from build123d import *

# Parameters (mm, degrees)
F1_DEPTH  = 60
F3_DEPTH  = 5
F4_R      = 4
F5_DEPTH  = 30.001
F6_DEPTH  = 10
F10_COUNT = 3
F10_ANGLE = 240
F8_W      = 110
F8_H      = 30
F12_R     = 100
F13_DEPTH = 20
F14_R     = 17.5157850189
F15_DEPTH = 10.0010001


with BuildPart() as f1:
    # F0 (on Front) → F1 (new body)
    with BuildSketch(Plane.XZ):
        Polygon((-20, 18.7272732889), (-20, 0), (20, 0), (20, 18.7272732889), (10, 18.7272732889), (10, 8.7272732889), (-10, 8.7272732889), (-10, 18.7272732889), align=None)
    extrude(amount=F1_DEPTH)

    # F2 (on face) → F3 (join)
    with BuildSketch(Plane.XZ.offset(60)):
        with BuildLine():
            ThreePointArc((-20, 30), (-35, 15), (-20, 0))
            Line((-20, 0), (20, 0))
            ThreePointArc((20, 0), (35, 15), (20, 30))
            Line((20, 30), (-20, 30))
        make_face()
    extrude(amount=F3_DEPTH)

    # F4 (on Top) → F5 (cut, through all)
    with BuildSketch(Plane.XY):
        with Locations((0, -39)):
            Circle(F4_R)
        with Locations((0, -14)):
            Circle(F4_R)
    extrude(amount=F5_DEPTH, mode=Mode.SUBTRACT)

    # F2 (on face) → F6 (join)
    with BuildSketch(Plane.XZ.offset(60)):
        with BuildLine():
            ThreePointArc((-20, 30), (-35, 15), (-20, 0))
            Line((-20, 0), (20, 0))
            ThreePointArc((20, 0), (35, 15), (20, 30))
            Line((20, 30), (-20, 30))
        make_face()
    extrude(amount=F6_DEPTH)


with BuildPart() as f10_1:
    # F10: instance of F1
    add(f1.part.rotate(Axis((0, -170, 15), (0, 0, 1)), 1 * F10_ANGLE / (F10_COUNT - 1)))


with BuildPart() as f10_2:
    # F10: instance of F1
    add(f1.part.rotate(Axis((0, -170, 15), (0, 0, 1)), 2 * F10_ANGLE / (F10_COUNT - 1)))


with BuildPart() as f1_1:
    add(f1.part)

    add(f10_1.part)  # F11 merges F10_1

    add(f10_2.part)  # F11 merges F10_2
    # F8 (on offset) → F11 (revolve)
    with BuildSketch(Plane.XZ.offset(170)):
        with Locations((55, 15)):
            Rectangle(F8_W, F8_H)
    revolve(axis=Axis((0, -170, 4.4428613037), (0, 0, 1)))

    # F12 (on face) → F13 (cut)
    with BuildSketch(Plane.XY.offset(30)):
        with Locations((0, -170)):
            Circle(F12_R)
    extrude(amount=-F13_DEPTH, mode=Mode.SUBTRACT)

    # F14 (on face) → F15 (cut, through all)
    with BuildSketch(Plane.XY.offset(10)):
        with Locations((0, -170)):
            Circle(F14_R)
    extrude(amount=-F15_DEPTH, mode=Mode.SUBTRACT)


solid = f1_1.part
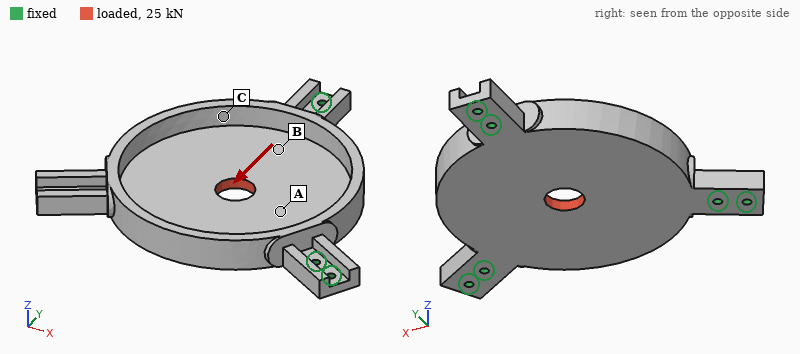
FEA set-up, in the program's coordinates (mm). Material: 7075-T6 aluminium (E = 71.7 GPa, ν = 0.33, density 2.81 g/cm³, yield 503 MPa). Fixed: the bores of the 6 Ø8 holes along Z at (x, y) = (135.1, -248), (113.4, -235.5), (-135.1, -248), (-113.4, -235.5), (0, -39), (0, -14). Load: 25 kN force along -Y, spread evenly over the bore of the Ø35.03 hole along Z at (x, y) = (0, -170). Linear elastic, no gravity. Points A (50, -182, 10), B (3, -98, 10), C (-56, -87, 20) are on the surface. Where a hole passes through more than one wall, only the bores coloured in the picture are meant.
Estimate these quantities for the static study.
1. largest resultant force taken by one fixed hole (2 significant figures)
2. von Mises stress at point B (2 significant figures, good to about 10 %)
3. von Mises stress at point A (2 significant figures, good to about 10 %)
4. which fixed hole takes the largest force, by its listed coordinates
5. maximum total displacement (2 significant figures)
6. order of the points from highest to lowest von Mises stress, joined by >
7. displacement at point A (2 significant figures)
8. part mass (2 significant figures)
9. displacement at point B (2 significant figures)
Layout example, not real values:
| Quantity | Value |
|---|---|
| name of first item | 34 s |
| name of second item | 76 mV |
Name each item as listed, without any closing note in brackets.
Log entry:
| Quantity | Value |
|---|---|
| largest resultant force taken by one fixed hole | 9.0 kN |
| von Mises stress at point B | 24 MPa |
| von Mises stress at point A | 10 MPa |
| which fixed hole takes the largest force, by its listed coordinates | (0, -39) |
| maximum total displacement | 49 µm |
| order of the points from highest to lowest von Mises stress, joined by > | B > A > C |
| displacement at point A | 31 µm |
| part mass | 1.7 kg |
| displacement at point B | 22 µm |
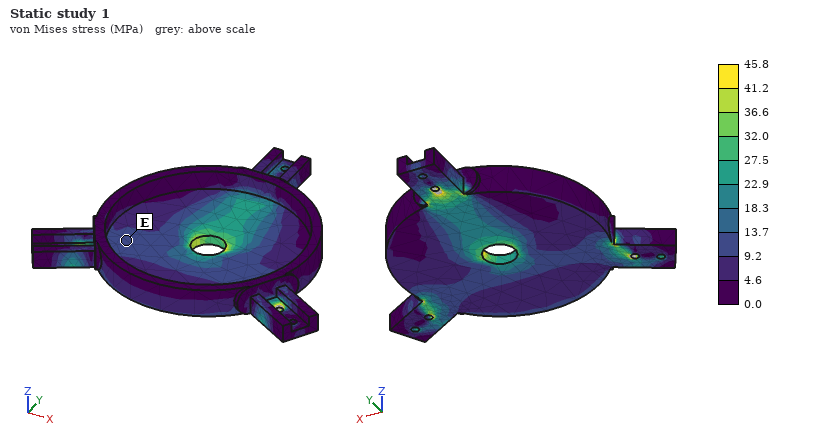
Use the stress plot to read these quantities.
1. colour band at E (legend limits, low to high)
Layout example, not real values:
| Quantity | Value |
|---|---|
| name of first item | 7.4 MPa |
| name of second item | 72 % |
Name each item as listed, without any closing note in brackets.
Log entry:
| Quantity | Value |
|---|---|
| colour band at E | 9.2 to 13.7 MPa |
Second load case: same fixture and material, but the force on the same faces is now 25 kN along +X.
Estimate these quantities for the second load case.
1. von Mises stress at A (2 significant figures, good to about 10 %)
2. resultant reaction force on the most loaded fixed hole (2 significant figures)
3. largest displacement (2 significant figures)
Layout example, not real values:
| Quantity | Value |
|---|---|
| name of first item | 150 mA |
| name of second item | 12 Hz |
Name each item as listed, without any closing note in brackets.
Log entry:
| Quantity | Value |
|---|---|
| von Mises stress at A | 20 MPa |
| resultant reaction force on the most loaded fixed hole | 8.4 kN |
| largest displacement | 49 µm |
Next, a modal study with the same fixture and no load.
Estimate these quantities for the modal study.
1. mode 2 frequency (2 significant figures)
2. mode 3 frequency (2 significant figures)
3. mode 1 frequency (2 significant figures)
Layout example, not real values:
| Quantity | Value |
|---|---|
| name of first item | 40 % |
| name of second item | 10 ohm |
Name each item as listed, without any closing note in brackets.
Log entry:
| Quantity | Value |
|---|---|
| mode 2 frequency | 1200 Hz |
| mode 3 frequency | 1200 Hz |
| mode 1 frequency | 1200 Hz |
